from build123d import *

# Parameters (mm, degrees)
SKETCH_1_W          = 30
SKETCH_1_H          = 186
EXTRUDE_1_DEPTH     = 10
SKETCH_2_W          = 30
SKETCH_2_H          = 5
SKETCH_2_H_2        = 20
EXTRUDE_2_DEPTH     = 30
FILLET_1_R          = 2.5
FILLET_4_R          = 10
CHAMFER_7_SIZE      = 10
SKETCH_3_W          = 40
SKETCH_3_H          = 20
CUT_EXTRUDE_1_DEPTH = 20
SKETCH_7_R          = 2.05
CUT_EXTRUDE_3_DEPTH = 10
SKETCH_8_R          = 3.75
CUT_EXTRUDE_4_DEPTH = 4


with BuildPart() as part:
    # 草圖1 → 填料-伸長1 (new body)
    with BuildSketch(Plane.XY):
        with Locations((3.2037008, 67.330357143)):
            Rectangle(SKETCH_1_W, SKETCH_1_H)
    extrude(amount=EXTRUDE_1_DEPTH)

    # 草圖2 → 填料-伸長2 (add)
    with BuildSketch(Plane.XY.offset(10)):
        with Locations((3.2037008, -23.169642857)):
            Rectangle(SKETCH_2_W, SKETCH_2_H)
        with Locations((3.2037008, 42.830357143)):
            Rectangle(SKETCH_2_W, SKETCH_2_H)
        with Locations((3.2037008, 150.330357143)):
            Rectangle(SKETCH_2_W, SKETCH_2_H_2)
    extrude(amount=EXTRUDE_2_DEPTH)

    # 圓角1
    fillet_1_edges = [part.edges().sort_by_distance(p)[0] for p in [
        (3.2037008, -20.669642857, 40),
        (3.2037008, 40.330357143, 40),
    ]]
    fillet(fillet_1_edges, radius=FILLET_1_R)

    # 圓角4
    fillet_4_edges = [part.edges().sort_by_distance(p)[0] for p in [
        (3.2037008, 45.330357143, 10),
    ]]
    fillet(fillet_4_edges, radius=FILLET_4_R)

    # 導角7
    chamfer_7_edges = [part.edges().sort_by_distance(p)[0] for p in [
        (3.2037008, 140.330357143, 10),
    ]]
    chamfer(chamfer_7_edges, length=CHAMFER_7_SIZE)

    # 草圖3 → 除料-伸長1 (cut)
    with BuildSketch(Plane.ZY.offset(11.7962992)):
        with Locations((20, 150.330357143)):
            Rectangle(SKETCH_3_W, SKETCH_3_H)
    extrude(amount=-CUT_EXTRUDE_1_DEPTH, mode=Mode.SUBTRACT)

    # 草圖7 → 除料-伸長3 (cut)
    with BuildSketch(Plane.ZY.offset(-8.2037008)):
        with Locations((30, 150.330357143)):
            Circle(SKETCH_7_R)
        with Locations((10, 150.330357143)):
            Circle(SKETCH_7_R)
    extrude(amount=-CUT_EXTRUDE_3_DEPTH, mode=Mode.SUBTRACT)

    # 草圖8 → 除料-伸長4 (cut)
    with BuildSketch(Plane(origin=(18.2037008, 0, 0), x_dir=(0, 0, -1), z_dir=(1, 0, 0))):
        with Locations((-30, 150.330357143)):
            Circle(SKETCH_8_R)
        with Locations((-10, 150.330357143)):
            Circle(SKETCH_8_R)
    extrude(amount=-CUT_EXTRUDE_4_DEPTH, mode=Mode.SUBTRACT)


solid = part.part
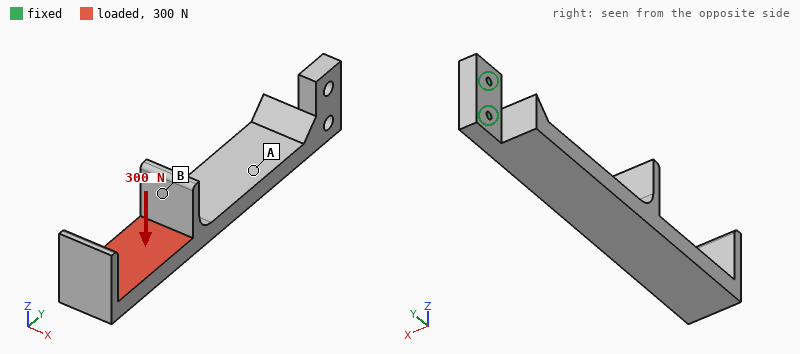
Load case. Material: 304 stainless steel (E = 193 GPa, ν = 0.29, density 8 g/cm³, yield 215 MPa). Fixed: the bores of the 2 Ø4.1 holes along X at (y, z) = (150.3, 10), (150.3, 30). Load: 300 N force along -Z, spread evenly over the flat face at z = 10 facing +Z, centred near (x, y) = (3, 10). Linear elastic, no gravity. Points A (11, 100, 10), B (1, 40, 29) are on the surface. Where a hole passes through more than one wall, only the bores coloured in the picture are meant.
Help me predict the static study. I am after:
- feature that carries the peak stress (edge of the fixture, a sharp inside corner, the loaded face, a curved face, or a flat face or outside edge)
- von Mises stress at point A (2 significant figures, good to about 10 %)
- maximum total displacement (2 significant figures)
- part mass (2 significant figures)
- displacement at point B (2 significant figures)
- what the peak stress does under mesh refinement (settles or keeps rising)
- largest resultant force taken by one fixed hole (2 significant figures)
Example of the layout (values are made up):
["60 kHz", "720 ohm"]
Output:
["edge of the fixture", "54 MPa", "0.78 mm", "550 g", "0.39 mm", "keeps rising", "2.0 kN"]
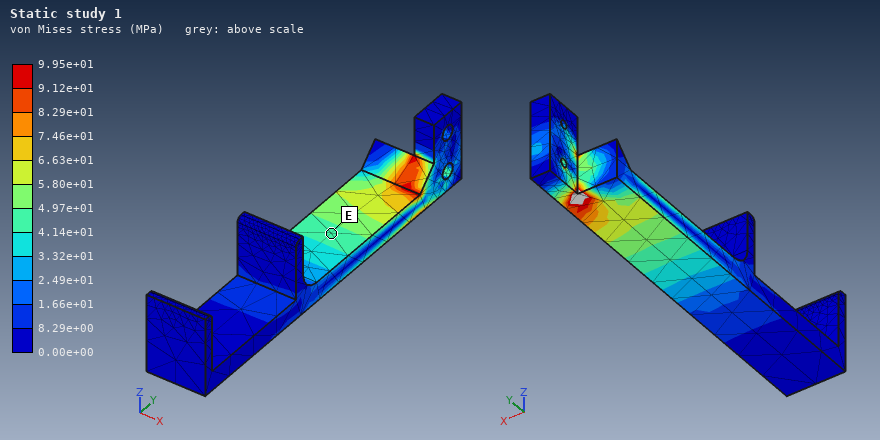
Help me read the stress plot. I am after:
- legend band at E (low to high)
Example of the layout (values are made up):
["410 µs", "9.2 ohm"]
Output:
["4.14e+01 to 4.97e+01 MPa"]
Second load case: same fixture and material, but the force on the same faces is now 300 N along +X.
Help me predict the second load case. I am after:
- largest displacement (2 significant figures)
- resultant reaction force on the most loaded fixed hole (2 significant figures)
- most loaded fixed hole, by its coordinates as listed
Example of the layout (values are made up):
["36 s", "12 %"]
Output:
["0.62 mm", "400 N", "(150.3, 10)"]
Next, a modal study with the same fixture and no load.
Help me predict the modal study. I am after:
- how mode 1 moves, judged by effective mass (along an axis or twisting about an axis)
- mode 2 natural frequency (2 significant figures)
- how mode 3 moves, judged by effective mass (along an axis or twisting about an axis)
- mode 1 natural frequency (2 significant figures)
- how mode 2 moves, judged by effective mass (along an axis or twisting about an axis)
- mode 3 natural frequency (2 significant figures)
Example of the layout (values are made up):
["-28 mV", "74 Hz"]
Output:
["along Z", "230 Hz", "along Z", "220 Hz", "along X", "1300 Hz"]
